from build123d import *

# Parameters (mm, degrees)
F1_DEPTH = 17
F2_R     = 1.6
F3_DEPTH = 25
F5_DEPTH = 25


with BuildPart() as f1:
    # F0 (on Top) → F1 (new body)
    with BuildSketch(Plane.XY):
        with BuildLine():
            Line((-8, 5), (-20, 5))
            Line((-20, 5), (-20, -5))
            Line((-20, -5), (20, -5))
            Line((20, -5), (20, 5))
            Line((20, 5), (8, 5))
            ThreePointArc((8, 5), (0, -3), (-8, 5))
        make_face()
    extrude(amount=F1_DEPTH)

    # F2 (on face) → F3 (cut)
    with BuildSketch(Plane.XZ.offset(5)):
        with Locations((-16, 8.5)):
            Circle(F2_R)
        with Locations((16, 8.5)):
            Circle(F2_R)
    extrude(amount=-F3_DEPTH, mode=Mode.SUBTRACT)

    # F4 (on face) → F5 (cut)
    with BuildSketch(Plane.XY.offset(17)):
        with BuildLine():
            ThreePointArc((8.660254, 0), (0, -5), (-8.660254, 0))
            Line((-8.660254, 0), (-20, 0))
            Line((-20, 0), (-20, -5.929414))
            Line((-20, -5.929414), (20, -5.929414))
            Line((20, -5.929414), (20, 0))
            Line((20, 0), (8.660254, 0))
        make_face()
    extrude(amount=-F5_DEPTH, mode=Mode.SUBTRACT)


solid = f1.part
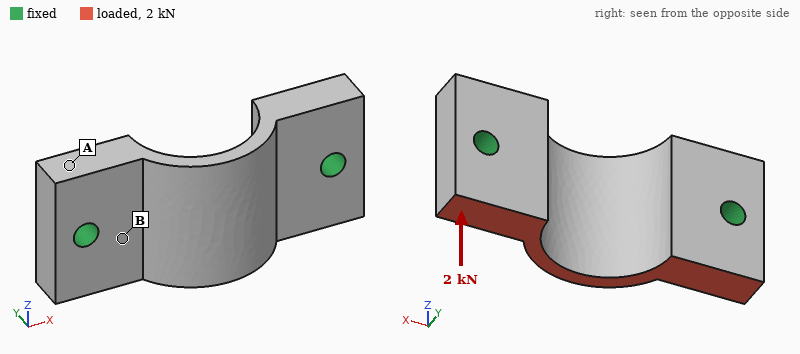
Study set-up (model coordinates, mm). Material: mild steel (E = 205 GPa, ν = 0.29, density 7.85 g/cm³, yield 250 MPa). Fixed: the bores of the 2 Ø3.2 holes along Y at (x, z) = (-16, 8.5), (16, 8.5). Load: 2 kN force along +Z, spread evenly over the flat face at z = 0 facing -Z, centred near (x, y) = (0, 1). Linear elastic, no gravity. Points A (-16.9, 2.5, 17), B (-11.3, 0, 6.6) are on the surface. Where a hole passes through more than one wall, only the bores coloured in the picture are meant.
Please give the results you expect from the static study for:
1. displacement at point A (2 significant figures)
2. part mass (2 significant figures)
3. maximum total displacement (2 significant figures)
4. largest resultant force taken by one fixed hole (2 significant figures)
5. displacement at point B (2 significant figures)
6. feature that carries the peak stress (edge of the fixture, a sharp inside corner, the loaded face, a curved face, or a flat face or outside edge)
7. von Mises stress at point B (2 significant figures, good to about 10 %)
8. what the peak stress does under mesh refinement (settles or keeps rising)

2.4 µm
21 g
9.1 µm
1.0 kN
2.2 µm
edge of the fixture
34 MPa
keeps rising
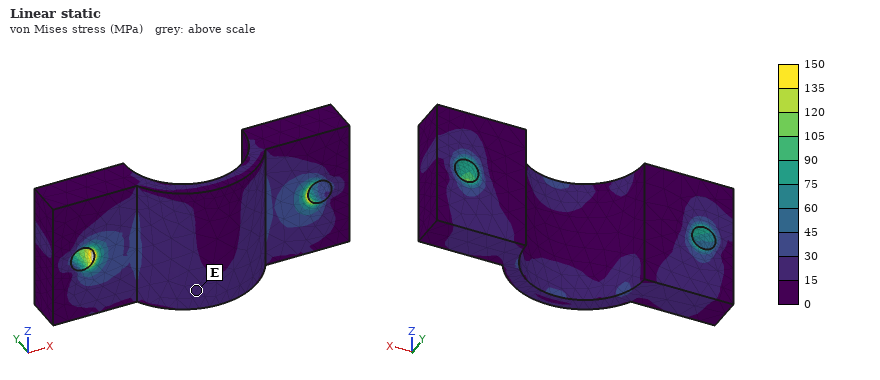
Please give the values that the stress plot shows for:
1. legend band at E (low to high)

15 to 30 MPa
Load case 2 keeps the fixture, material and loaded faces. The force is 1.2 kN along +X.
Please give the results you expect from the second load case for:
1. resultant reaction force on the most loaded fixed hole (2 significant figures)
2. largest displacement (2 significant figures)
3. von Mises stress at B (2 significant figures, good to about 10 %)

630 N
4.1 µm
24 MPa
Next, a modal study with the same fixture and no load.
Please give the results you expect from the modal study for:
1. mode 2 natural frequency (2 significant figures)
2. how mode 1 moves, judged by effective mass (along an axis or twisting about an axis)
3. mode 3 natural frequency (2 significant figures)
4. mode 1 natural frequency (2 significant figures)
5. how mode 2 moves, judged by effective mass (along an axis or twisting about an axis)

30 kHz
along Z
32 kHz
19 kHz
along Y
